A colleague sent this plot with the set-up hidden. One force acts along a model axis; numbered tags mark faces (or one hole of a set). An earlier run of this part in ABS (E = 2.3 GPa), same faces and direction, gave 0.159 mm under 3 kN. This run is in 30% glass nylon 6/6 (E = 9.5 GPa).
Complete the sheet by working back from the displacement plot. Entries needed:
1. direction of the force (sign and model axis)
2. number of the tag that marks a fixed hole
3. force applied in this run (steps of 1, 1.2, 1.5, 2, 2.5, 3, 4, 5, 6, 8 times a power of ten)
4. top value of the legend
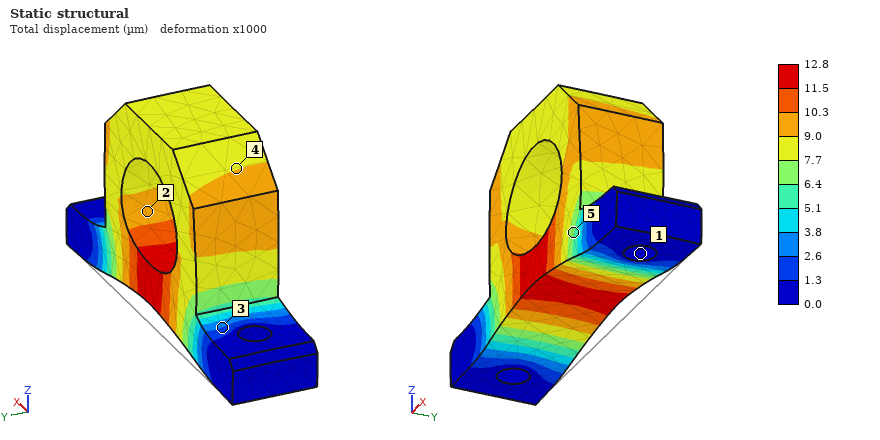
+Z
1
1 kN
12.8 µm
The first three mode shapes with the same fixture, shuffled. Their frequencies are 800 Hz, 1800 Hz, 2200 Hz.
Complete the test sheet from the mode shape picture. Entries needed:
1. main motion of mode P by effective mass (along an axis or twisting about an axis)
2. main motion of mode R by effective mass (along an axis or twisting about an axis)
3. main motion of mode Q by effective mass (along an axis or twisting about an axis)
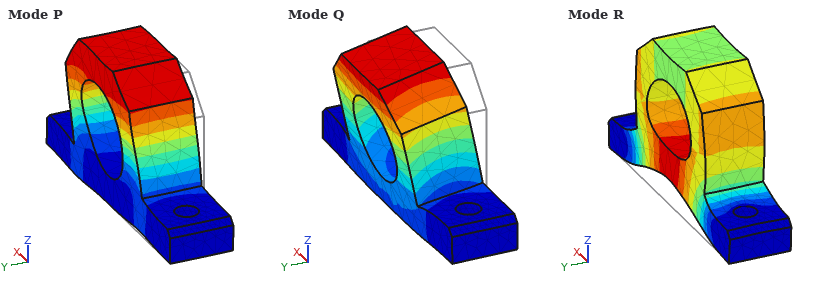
along X
along Z
along Y
